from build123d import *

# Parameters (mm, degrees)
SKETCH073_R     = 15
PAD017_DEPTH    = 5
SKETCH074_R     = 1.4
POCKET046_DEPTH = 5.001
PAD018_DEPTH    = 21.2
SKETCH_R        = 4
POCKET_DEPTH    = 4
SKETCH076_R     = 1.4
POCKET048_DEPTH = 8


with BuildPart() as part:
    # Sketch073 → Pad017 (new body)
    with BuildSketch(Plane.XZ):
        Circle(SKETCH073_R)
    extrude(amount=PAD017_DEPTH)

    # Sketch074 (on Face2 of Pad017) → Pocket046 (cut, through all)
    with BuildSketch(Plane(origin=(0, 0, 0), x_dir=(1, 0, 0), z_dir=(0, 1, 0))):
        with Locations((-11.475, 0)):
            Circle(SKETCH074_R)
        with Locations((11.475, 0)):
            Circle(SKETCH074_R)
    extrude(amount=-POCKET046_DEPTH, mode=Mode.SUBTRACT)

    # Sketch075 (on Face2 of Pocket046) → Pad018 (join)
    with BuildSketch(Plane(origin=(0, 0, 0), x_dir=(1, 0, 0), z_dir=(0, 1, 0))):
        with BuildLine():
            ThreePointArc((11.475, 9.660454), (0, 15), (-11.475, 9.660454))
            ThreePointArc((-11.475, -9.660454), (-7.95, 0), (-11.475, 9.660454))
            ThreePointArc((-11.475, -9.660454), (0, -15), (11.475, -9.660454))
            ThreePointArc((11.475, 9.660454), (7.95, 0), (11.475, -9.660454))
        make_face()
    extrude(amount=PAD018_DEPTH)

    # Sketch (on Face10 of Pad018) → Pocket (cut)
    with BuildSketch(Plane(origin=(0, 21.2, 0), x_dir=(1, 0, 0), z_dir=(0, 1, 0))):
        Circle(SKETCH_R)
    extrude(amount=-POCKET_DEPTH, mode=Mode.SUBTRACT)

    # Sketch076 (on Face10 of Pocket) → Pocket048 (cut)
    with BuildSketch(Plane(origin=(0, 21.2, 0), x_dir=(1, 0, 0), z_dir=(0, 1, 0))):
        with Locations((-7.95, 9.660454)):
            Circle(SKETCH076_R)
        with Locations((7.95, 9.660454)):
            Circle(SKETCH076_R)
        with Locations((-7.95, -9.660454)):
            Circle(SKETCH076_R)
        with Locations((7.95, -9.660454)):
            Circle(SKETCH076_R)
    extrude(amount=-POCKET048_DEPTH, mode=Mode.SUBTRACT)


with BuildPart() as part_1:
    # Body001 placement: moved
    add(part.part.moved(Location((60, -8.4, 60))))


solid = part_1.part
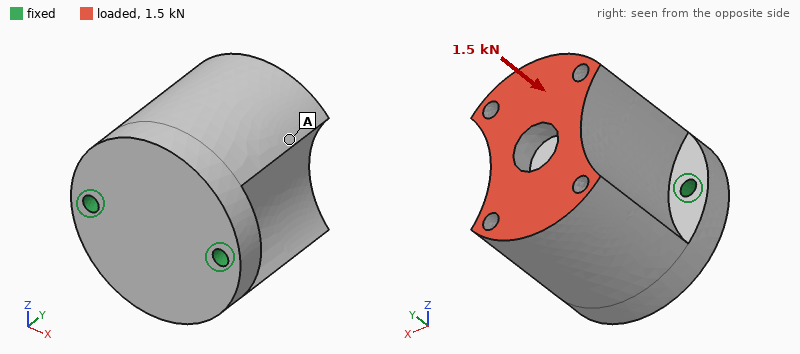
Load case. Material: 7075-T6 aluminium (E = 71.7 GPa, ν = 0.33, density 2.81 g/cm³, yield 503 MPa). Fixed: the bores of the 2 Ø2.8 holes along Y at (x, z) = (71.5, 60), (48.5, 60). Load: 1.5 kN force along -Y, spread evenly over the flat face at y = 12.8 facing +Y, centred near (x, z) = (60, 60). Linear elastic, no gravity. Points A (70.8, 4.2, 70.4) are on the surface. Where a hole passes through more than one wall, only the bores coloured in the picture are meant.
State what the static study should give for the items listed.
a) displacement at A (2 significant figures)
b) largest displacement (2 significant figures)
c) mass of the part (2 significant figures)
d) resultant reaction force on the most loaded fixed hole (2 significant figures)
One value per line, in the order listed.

4.5 µm
4.9 µm
40 g
780 N
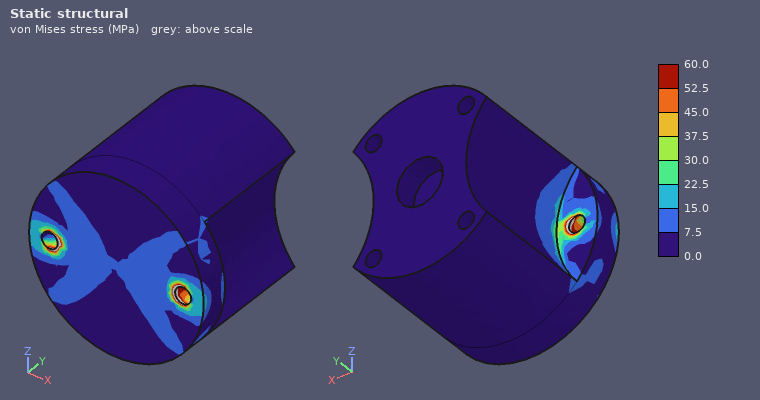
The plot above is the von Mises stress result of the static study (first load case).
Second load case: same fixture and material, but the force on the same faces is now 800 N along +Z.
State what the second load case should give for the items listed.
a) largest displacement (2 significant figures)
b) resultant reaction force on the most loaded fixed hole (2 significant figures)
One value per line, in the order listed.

89 µm
400 N
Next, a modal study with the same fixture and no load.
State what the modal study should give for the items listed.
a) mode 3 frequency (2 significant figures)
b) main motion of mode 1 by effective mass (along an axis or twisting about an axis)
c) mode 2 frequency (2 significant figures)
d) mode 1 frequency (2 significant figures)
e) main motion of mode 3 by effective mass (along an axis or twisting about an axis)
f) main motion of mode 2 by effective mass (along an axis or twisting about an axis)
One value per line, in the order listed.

16 kHz
along Z
11 kHz
4200 Hz
along Y
along X
